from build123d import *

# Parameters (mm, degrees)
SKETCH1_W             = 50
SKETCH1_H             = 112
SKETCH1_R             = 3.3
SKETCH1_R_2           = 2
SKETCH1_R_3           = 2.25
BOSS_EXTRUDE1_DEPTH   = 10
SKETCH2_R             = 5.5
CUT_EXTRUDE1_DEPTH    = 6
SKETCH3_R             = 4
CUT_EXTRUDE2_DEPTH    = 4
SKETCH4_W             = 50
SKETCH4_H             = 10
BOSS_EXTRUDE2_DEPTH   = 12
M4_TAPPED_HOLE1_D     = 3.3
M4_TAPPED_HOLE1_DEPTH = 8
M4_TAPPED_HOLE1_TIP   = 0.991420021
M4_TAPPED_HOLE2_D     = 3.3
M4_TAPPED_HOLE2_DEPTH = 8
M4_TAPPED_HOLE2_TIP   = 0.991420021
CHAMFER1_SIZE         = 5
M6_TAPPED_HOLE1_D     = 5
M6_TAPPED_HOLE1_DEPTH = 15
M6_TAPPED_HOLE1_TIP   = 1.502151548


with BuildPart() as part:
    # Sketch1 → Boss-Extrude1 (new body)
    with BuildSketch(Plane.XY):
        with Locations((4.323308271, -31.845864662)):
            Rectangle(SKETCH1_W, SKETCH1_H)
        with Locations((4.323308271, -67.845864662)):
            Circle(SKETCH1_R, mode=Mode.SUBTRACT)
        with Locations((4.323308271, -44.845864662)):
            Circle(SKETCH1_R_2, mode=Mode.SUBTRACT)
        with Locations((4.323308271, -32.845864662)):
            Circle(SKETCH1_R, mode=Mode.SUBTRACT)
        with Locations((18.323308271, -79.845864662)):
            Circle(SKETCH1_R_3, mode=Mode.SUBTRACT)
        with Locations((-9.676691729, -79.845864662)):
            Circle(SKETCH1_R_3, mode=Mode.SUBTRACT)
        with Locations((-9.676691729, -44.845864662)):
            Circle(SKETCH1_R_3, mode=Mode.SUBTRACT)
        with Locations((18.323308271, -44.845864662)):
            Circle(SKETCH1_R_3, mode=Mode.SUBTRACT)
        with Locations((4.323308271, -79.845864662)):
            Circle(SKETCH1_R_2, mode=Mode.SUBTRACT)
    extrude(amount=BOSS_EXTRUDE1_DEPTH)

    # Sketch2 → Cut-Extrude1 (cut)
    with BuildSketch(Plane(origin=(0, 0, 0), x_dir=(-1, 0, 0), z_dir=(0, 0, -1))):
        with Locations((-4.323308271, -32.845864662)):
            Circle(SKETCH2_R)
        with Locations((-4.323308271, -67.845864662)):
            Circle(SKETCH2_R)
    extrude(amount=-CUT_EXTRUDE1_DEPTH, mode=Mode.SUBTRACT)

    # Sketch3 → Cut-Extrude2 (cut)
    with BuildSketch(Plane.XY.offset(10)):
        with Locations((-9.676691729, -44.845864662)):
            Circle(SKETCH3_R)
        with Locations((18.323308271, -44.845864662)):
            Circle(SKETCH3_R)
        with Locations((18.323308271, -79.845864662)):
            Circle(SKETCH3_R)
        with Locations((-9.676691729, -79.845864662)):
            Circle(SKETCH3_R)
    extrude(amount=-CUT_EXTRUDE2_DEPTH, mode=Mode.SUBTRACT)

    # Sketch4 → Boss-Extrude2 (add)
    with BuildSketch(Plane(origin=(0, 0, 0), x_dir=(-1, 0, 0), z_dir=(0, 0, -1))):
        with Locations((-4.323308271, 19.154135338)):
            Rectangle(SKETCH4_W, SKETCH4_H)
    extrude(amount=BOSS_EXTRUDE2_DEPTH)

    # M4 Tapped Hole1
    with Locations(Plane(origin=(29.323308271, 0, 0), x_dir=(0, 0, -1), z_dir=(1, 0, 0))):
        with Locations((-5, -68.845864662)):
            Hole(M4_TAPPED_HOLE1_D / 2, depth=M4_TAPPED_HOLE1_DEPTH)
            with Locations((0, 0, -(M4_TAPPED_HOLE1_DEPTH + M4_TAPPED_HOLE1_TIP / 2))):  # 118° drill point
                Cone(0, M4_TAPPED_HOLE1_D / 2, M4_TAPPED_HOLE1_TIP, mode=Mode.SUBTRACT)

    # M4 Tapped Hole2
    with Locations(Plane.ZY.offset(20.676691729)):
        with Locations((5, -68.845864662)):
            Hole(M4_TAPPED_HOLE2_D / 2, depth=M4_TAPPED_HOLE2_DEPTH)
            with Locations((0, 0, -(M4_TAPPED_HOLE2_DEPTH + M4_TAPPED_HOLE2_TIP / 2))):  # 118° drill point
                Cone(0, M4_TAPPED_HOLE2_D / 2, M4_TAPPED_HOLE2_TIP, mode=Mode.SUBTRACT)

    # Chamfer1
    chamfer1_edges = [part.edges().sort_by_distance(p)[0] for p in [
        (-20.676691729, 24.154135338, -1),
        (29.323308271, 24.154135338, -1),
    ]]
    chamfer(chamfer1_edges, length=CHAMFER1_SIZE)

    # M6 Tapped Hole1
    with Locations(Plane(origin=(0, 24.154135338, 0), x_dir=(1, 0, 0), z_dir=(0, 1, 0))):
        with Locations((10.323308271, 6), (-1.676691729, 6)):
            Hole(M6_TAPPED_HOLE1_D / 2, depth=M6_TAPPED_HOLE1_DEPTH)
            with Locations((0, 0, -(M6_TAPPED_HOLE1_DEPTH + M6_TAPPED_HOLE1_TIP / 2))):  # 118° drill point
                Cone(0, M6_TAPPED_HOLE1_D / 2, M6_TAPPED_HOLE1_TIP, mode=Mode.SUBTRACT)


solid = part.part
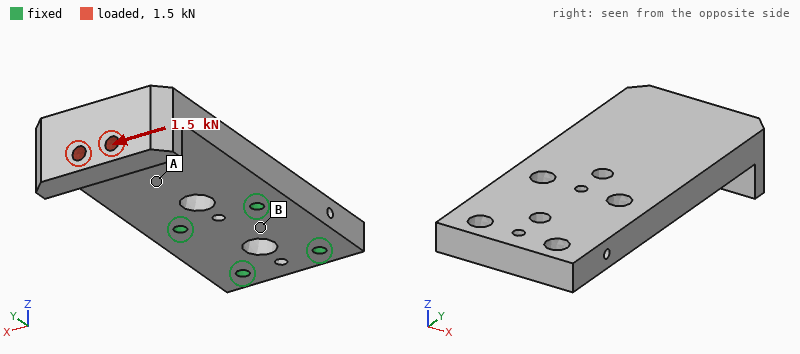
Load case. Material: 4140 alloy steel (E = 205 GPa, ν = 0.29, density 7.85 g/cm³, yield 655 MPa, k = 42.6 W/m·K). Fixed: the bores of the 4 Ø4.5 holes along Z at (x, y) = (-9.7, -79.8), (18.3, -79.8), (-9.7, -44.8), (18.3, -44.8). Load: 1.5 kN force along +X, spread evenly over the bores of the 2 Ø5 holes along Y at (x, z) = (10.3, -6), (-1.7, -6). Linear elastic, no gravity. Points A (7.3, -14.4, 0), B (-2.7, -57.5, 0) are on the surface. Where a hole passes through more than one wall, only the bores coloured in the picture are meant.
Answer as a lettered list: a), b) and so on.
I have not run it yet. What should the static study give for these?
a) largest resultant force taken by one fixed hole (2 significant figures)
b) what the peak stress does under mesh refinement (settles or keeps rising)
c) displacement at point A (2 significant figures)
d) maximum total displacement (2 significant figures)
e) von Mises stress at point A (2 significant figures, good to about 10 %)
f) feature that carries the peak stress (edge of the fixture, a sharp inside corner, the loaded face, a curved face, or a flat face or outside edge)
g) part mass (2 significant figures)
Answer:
a) 2.3 kN
b) keeps rising
c) 7.4 µm
d) 34 µm
e) 28 MPa
f) edge of the fixture
g) 460 g
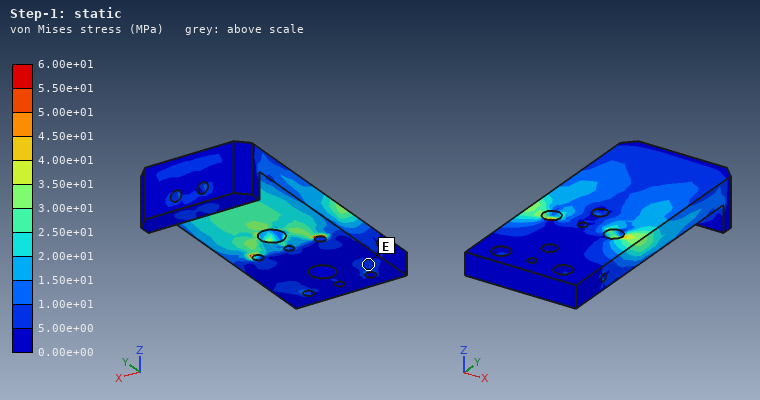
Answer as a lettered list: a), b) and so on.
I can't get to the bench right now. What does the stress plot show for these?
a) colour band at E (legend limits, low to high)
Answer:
a) 5.00e+00 to 1.00e+01 MPa
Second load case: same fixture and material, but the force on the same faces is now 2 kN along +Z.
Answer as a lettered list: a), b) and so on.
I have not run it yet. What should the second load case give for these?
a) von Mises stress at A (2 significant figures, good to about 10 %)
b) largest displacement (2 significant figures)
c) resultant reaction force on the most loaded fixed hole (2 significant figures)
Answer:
a) 71 MPa
b) 0.33 mm
c) 2.8 kN
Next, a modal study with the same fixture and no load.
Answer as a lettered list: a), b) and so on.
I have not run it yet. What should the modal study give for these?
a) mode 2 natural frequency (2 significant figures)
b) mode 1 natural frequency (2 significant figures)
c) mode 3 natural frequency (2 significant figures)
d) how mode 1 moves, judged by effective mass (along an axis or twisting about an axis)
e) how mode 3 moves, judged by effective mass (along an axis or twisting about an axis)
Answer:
a) 3600 Hz
b) 1200 Hz
c) 4900 Hz
d) along Z
e) along X
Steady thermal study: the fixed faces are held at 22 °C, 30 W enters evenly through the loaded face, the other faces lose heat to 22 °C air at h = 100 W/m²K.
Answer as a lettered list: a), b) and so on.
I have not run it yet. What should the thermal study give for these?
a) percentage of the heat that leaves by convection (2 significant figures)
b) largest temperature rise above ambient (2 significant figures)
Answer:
a) 76 %
b) 57 K
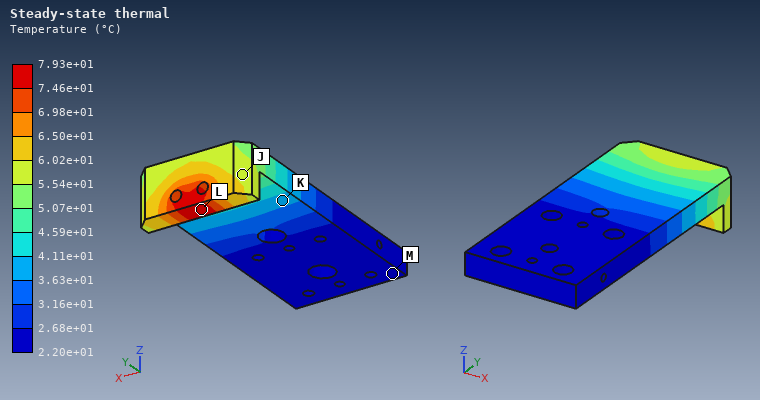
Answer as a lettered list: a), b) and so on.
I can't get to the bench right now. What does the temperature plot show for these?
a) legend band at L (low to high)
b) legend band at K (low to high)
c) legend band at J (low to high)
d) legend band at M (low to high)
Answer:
a) 7.46e+01 to 7.93e+01 °C
b) 3.63e+01 to 4.11e+01 °C
c) 5.54e+01 to 6.02e+01 °C
d) 2.20e+01 to 2.68e+01 °C
